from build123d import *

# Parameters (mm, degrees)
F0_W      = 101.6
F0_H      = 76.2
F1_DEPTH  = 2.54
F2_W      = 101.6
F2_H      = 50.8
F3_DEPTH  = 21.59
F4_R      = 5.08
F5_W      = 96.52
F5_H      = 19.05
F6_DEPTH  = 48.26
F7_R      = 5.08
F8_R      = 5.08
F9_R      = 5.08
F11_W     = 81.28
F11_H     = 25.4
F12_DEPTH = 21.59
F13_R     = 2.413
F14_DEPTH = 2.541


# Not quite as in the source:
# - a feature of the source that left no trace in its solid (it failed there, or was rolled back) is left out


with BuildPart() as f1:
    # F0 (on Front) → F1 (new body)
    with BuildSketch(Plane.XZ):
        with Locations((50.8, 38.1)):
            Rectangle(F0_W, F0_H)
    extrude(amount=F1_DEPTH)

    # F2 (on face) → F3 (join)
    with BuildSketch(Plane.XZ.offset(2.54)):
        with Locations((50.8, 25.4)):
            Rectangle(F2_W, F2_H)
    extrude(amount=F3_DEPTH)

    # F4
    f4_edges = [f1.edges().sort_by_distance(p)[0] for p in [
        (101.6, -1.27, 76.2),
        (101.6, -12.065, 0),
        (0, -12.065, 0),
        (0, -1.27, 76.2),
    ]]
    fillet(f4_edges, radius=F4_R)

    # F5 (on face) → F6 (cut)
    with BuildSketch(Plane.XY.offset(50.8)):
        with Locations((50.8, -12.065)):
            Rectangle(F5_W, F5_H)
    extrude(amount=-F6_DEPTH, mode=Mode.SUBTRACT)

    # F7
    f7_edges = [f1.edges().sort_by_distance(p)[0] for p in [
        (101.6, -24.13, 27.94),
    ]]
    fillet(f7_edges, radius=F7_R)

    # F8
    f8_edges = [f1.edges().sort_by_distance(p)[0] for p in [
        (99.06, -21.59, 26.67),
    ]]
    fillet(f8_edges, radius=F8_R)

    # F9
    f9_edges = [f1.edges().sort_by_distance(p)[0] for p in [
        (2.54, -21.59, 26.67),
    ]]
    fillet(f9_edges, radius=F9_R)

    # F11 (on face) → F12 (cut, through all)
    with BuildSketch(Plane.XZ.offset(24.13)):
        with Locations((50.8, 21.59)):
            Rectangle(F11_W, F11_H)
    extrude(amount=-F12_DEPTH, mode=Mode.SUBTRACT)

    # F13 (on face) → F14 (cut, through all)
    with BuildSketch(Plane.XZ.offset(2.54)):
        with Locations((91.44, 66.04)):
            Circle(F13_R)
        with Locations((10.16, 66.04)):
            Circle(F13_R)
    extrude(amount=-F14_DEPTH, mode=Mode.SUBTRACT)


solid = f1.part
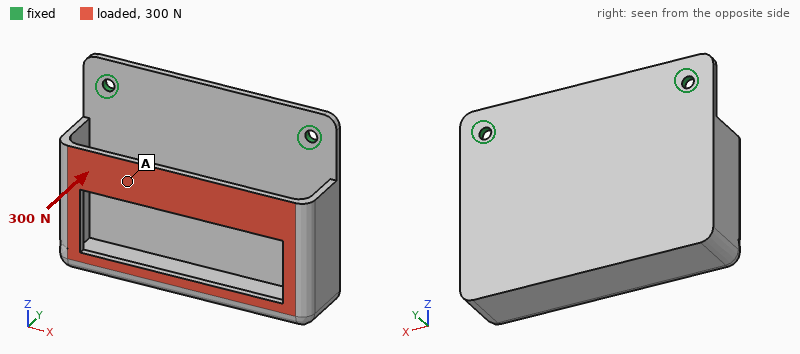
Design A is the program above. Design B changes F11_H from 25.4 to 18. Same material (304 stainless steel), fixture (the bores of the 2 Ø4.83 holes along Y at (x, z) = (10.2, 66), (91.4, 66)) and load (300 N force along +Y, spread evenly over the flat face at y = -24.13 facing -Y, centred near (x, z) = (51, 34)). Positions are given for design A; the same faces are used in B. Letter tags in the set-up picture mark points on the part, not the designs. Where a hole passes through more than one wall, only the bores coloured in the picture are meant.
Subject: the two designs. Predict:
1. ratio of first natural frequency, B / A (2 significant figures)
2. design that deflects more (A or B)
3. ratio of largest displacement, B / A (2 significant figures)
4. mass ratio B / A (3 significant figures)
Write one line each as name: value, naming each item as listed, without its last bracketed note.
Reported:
ratio of first natural frequency, B / A: 0.97
design that deflects more: B
ratio of largest displacement, B / A: 1.1
mass ratio B / A: 1.04
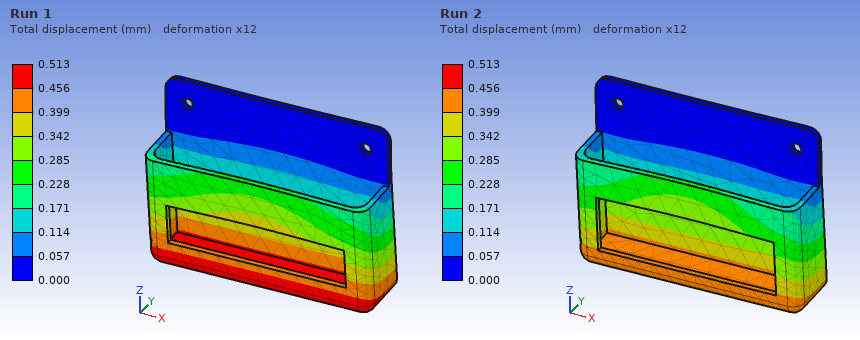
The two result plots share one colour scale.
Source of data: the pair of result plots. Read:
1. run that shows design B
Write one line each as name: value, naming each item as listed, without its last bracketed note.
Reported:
run that shows design B: Run 1
